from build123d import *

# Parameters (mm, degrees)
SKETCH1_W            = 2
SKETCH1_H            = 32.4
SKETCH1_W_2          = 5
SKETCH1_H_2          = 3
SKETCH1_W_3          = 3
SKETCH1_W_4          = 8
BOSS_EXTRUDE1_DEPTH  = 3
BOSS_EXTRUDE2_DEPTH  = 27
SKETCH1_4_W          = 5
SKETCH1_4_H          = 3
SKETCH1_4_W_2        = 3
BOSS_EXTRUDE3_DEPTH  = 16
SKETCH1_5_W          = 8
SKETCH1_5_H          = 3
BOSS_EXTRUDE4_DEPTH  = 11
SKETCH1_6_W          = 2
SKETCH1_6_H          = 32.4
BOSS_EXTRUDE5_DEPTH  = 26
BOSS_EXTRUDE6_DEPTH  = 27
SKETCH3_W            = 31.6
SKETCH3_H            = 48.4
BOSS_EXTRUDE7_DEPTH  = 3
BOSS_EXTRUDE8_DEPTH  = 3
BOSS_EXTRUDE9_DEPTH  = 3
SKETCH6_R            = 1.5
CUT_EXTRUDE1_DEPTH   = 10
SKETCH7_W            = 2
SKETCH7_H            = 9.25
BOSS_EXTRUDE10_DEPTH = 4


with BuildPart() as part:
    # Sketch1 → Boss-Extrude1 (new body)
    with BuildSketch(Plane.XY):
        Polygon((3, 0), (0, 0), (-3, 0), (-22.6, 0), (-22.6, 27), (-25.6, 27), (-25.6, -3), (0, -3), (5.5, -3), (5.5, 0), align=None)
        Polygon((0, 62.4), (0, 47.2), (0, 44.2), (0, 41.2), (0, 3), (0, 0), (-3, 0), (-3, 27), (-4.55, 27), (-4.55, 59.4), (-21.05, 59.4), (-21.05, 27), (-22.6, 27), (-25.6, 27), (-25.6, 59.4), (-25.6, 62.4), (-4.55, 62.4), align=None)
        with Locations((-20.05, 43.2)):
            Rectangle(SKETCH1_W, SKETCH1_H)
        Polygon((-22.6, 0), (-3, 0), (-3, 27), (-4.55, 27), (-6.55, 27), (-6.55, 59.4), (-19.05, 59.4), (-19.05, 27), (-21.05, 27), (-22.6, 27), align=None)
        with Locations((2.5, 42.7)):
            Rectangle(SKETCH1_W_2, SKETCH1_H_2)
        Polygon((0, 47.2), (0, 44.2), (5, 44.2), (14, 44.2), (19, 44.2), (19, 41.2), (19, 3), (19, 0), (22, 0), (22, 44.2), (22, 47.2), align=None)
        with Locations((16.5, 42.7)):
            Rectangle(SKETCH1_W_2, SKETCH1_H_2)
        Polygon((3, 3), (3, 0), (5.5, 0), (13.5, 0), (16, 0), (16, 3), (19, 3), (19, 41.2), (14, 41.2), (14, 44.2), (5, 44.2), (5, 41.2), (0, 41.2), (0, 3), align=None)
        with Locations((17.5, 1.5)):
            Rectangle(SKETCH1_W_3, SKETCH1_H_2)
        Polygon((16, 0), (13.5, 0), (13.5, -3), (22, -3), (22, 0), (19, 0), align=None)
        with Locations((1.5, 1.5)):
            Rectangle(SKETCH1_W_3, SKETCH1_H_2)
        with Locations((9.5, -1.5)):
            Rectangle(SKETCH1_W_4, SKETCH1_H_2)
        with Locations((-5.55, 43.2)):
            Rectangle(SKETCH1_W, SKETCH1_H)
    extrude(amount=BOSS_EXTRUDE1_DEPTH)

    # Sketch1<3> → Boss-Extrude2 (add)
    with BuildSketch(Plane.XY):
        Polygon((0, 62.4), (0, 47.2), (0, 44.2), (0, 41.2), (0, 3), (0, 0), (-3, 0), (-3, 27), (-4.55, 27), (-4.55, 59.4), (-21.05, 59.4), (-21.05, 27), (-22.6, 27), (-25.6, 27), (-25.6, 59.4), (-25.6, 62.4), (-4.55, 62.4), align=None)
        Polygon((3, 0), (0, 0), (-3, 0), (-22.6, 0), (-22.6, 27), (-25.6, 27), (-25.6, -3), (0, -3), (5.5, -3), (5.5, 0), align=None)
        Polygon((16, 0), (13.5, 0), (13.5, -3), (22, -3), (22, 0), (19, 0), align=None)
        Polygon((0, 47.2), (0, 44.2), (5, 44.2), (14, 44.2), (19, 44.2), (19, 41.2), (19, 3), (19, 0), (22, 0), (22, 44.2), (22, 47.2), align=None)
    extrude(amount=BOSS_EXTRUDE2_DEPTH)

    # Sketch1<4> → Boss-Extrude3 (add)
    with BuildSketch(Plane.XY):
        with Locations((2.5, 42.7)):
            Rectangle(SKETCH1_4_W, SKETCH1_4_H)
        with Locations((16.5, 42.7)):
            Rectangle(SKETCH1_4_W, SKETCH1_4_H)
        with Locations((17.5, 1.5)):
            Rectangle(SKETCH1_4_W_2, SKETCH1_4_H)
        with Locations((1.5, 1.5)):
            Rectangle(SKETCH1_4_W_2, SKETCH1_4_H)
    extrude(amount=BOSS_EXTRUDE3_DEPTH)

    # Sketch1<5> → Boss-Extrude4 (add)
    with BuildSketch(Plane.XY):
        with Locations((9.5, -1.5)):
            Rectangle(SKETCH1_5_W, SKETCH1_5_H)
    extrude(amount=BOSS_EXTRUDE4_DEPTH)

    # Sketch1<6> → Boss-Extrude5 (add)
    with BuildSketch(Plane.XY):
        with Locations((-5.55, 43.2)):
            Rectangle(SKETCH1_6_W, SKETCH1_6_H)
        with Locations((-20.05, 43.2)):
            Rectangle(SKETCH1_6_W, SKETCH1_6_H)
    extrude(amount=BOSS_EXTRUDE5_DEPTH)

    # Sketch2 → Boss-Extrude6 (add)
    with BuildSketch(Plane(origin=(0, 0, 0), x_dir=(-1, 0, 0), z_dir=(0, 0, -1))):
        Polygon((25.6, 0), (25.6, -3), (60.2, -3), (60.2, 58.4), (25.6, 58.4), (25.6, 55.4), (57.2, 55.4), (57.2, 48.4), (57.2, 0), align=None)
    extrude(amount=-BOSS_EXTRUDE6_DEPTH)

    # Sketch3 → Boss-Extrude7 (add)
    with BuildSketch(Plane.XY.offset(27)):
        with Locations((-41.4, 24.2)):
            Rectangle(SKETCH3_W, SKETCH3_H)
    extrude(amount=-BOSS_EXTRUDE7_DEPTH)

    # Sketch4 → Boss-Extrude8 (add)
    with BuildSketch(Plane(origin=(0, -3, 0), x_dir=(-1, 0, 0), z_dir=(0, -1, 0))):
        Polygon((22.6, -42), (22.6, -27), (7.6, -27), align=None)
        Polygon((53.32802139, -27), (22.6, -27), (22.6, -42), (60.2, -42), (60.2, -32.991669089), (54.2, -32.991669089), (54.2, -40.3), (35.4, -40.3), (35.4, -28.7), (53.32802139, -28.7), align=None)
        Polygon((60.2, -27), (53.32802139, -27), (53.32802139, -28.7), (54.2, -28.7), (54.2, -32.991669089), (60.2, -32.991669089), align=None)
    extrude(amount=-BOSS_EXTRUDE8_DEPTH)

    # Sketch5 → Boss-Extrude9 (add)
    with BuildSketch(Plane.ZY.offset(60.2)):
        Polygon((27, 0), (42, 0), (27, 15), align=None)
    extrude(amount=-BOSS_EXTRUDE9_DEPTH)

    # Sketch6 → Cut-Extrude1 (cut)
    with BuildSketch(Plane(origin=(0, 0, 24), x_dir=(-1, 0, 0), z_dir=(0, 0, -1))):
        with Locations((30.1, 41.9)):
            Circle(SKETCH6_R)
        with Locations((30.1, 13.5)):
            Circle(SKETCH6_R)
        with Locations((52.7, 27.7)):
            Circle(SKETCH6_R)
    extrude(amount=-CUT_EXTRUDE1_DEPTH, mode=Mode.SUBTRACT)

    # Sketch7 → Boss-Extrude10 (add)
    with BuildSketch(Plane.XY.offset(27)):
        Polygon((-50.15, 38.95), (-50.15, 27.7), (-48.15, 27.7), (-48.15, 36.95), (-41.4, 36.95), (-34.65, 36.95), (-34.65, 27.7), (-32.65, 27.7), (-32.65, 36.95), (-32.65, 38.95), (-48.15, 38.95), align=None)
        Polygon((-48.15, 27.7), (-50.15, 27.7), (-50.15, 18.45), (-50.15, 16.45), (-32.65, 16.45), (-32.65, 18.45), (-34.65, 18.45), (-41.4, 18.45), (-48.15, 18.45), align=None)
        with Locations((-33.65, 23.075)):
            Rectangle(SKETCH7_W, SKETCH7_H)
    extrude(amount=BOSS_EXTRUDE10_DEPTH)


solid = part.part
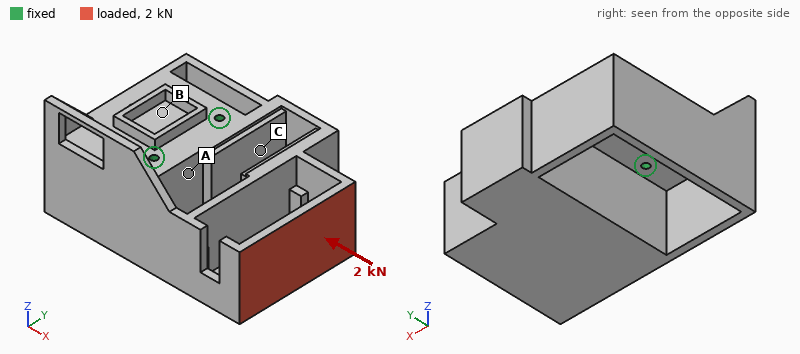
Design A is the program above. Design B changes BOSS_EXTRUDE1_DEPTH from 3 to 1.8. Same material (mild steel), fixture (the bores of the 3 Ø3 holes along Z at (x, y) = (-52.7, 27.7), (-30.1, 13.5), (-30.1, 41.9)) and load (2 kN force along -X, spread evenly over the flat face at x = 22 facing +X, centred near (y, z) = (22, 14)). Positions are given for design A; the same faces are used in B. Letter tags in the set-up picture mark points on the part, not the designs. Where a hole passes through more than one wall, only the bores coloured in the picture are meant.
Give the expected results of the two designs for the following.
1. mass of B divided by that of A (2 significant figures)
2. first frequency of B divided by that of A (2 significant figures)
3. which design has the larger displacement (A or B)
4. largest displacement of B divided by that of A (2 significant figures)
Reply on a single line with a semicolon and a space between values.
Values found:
0.96; 1.0; B; 1.1
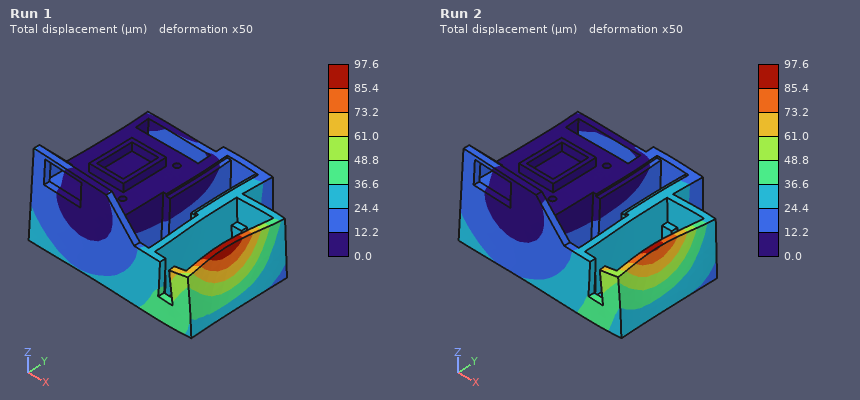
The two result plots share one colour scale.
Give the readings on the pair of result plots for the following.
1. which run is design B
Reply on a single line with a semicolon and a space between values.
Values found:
Run 1
